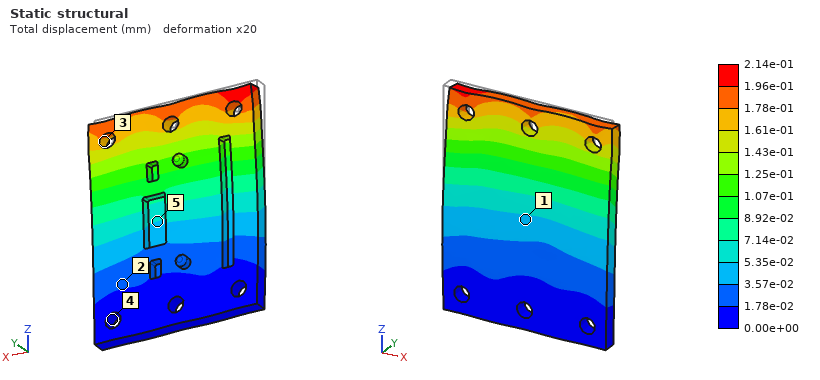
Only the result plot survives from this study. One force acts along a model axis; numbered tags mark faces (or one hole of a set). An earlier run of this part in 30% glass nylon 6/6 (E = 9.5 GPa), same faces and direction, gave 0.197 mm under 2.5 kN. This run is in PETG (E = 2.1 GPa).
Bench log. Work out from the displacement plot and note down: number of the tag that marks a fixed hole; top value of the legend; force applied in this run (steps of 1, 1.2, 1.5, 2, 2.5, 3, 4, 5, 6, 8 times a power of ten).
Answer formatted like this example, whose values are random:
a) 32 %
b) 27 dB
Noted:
a) 4
b) 2.14e-01 mm
c) 600 N
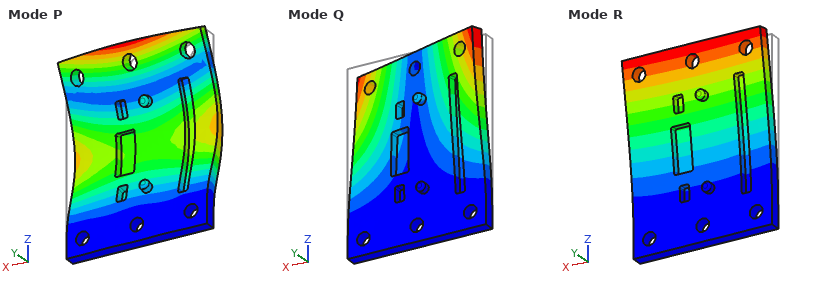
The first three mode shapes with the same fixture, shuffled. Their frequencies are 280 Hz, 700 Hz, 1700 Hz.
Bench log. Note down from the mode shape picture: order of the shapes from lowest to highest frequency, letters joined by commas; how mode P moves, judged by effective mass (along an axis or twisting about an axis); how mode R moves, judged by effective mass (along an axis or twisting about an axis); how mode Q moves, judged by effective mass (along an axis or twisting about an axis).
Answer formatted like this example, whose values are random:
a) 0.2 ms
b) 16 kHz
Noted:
a) R, Q, P
b) along Y
c) along Y
d) twisting about Z
